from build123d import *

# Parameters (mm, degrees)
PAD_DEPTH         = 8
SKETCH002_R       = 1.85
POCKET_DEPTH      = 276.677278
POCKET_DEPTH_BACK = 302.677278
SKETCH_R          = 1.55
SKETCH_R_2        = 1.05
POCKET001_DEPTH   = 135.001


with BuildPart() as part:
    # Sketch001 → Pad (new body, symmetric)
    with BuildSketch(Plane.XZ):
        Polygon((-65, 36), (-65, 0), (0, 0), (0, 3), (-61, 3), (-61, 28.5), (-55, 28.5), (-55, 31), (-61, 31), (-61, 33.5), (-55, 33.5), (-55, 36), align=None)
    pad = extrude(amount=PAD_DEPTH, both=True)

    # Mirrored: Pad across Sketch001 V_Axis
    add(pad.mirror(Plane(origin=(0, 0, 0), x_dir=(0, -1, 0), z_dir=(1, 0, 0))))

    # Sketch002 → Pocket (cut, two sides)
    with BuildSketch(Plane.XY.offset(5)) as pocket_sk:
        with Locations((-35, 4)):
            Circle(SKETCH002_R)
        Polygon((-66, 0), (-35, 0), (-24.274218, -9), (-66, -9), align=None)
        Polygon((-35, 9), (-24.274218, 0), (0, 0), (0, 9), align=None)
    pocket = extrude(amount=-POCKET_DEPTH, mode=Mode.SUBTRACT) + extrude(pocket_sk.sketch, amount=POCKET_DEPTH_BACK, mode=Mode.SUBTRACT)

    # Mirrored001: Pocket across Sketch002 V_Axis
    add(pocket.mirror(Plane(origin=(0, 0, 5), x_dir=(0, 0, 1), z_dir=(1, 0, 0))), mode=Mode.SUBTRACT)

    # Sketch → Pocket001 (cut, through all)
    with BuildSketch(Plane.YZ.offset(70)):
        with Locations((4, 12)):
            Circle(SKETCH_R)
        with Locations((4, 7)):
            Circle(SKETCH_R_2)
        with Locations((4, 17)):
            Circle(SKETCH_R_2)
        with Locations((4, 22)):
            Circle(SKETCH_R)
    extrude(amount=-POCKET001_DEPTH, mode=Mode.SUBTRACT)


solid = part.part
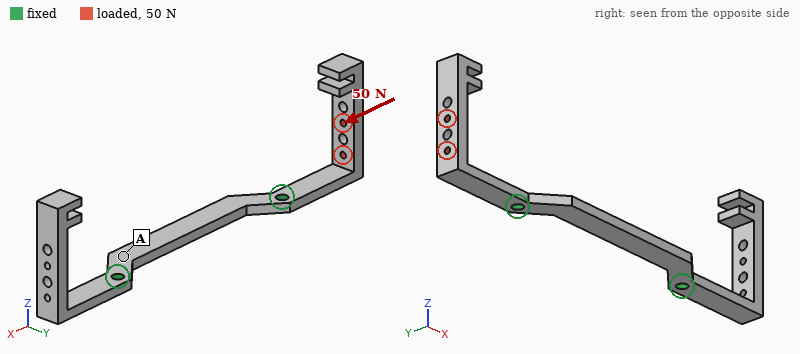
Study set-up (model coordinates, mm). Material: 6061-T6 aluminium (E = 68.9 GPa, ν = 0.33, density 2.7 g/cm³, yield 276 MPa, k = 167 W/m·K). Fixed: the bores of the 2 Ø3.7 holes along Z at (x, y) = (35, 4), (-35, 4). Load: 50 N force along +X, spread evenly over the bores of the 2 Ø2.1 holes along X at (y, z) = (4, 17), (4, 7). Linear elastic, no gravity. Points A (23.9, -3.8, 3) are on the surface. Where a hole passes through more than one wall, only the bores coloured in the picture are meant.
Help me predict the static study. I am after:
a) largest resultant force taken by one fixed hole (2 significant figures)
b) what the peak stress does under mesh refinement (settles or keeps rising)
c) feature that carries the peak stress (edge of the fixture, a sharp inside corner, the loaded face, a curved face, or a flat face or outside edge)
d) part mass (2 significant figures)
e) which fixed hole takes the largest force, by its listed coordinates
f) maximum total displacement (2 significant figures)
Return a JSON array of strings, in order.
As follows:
["50 N", "keeps rising", "edge of the fixture", "15 g", "(-35, 4)", "0.45 mm"]
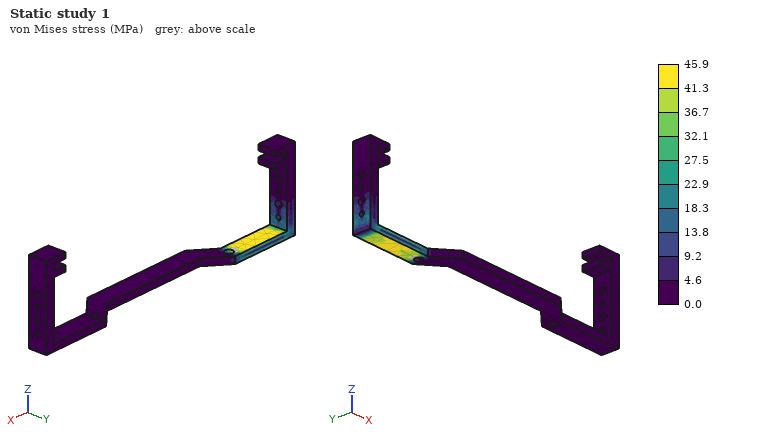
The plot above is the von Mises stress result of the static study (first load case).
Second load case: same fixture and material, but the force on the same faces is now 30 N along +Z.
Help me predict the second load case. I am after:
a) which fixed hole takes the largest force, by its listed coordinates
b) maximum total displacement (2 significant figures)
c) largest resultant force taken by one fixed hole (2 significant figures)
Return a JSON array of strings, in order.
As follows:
["(-35, 4)", "0.34 mm", "30 N"]
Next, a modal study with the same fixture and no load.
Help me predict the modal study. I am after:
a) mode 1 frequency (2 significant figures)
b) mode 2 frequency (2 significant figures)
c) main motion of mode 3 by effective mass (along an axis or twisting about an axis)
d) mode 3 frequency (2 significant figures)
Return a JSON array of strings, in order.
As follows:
["680 Hz", "680 Hz", "along Y", "870 Hz"]
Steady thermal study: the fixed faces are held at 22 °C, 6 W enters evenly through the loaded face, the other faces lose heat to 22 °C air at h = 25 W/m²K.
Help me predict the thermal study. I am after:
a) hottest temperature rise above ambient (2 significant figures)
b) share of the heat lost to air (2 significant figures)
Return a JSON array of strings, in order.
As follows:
["41 K", "22 %"]
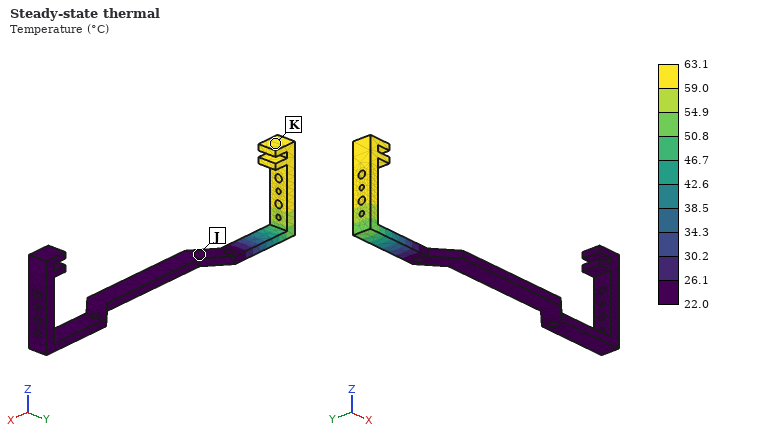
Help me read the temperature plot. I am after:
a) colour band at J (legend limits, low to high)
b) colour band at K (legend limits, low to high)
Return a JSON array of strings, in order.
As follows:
["22.0 to 26.1 °C", "59.0 to 63.1 °C"]
